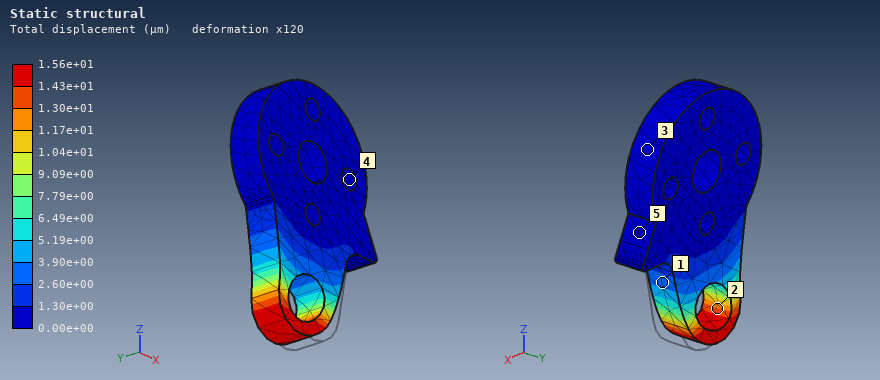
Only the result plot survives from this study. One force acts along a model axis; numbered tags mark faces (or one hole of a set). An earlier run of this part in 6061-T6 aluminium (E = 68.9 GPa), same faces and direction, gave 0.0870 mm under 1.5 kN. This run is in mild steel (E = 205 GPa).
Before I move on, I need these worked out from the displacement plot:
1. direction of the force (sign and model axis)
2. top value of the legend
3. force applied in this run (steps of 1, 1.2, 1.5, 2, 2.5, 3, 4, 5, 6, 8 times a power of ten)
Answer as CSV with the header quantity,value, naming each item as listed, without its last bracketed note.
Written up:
quantity,value
direction of the force,-X
top value of the legend,1.56e+01 µm
force applied in this run,800 N
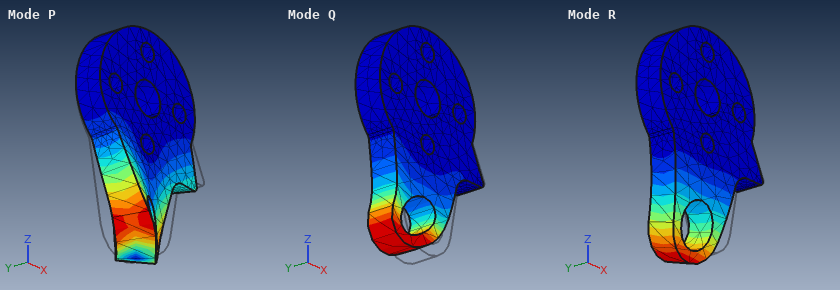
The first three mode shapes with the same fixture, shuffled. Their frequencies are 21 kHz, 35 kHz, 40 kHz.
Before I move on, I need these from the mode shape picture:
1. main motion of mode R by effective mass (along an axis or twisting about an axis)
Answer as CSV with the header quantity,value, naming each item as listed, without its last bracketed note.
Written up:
quantity,value
main motion of mode R by effective mass,along Y
